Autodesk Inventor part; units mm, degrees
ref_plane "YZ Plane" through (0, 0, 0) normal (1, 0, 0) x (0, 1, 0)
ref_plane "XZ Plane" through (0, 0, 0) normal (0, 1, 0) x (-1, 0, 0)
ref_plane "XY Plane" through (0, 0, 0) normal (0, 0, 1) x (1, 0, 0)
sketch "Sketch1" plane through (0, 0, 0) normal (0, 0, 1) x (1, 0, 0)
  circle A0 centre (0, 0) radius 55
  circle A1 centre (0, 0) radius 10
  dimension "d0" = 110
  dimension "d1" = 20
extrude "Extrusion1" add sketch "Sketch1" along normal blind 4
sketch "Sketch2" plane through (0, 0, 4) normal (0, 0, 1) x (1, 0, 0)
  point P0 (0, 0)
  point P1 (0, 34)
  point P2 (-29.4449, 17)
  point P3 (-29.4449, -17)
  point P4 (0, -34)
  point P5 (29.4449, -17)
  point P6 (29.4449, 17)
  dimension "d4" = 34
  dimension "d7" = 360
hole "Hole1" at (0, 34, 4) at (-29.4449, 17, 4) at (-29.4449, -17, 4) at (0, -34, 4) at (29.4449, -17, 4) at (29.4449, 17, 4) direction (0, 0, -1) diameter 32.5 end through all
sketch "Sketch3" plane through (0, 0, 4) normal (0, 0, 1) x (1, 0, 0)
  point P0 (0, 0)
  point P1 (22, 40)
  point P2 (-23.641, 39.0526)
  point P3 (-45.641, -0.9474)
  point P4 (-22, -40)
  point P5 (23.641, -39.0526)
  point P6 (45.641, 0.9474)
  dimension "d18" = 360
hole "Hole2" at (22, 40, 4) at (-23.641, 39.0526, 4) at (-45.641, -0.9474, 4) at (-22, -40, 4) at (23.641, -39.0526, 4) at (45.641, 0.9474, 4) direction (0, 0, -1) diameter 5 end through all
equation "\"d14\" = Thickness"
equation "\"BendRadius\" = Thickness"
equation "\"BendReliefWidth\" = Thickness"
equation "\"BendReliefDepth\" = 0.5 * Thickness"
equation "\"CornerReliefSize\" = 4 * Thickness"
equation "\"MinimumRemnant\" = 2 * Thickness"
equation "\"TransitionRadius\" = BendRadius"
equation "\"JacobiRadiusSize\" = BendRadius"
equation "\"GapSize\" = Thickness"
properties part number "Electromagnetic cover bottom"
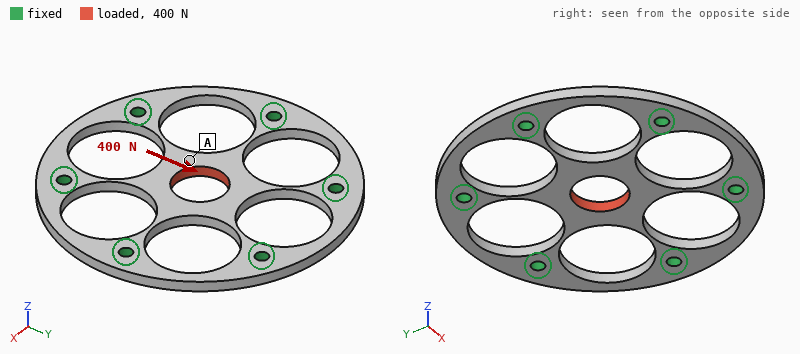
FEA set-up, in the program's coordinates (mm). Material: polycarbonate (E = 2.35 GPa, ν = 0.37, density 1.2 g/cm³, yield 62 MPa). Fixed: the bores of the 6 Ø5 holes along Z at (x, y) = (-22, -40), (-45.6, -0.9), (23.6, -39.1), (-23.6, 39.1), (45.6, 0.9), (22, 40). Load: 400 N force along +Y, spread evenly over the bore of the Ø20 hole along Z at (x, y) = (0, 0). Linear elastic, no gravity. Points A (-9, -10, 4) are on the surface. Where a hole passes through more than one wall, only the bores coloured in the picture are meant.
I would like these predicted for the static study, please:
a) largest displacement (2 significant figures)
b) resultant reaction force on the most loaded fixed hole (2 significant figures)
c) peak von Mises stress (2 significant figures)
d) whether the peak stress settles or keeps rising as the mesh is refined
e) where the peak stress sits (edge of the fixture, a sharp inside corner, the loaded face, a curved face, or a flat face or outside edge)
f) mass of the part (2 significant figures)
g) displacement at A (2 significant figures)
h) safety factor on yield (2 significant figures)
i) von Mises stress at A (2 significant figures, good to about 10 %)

0.12 mm
110 N
20 MPa
settles
a curved face
20 g
0.12 mm
3.0
2.4 MPa
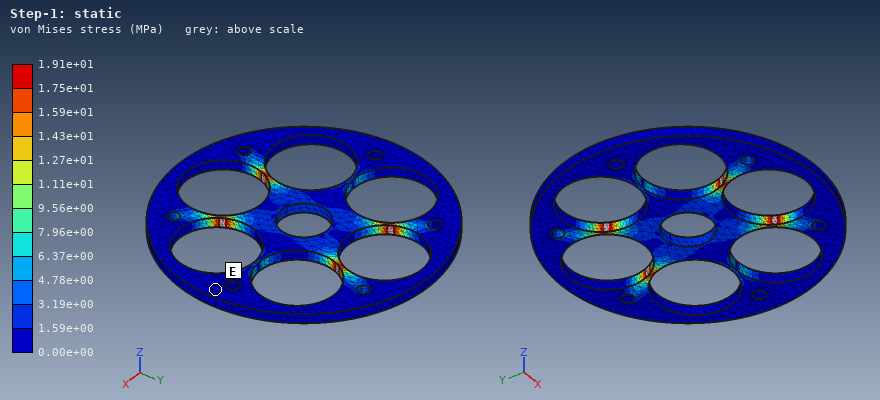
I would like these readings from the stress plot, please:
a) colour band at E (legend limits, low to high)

0.00e+00 to 1.59e+00 MPa
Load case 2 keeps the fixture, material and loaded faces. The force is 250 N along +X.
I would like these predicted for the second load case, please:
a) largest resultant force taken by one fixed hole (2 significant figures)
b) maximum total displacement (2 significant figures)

78 N
77 µm
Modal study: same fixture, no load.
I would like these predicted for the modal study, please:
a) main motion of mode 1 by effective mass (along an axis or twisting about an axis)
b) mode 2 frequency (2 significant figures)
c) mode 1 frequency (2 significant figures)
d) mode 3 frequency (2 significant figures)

along Z
1800 Hz
870 Hz
1800 Hz
